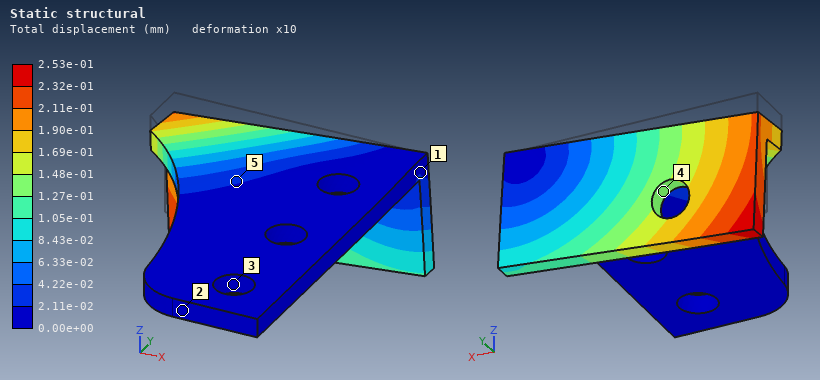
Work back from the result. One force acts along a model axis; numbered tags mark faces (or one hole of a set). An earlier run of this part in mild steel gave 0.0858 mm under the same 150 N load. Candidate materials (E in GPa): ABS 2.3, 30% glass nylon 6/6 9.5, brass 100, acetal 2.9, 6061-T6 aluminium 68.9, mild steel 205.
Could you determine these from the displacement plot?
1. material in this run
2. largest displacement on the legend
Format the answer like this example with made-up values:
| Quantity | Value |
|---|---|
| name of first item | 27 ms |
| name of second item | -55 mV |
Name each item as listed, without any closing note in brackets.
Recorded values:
| Quantity | Value |
|---|---|
| material in this run | 6061-T6 aluminium |
| largest displacement on the legend | 2.53e-01 mm |
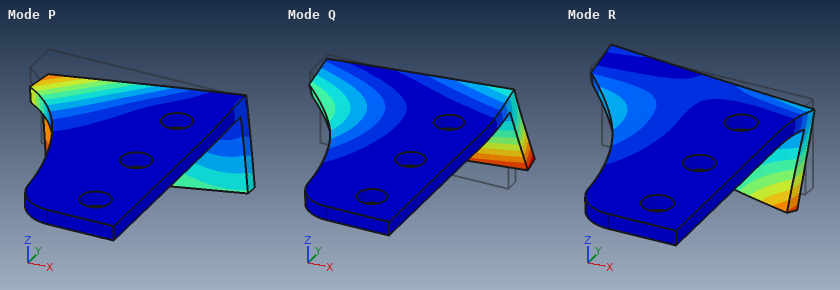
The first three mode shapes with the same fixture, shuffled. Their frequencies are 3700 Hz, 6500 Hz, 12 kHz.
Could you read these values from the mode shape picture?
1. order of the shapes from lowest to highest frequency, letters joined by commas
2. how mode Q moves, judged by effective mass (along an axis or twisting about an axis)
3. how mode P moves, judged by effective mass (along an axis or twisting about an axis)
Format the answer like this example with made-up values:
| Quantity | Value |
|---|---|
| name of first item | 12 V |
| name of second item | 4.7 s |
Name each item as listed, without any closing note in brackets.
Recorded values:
| Quantity | Value |
|---|---|
| order of the shapes from lowest to highest frequency, letters joined by commas | P, Q, R |
| how mode Q moves, judged by effective mass | along Y |
| how mode P moves, judged by effective mass | along Z |
